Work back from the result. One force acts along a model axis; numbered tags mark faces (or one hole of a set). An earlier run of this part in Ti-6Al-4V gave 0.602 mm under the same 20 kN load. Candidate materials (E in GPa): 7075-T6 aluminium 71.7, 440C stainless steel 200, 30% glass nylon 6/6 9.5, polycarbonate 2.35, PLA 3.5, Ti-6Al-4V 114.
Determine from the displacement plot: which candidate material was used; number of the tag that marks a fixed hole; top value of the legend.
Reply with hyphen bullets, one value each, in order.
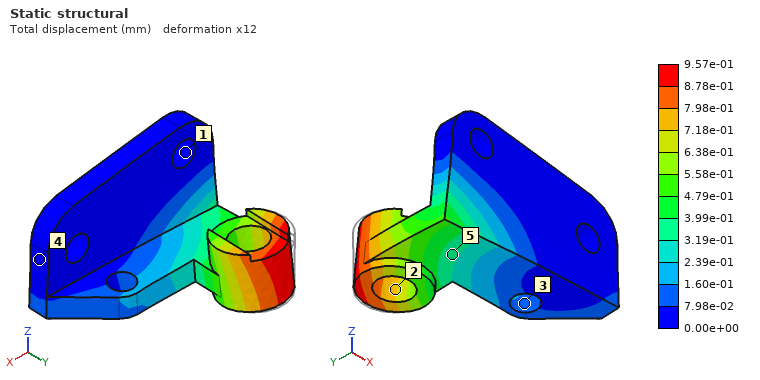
- 7075-T6 aluminium
- 1
- 9.57e-01 mm
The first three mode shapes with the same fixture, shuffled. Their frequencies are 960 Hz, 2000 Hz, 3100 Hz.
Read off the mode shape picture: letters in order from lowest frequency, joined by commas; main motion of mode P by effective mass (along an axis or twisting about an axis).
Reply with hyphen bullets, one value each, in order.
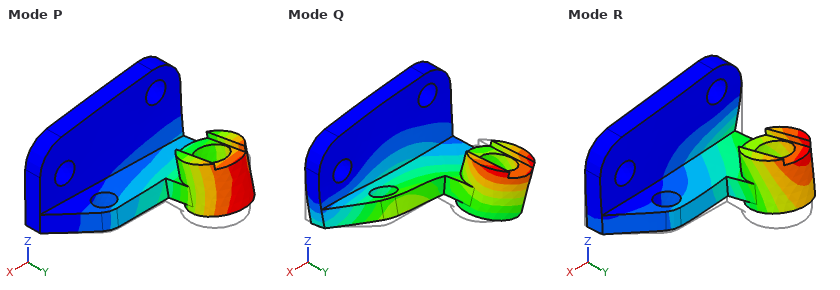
- P, R, Q
- along Z
